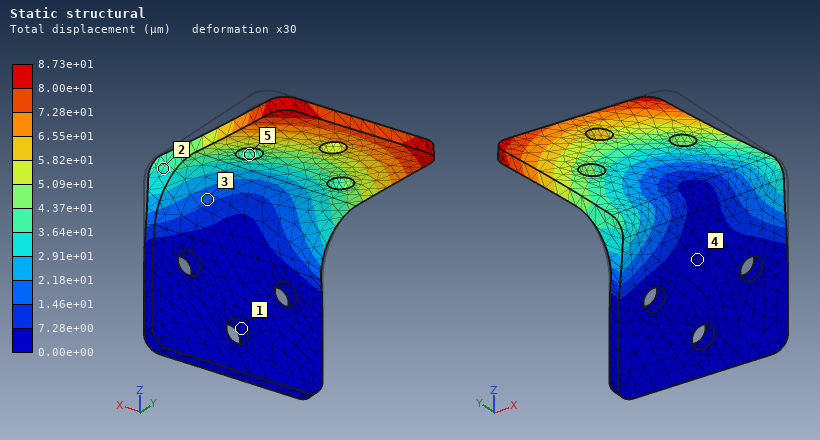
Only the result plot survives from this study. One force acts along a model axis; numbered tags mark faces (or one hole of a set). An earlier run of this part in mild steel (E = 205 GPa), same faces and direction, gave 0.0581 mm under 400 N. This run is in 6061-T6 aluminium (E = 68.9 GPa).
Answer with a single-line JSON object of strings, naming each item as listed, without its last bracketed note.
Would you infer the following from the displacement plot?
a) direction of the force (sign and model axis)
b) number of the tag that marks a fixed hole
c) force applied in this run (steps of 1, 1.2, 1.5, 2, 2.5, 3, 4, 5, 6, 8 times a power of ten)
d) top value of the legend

{"direction of the force": "-X", "number of the tag that marks a fixed hole": "1", "force applied in this run": "200 N", "top value of the legend": "8.73e+01 µm"}
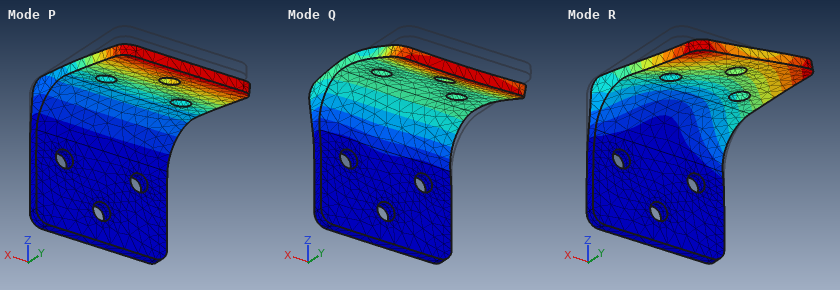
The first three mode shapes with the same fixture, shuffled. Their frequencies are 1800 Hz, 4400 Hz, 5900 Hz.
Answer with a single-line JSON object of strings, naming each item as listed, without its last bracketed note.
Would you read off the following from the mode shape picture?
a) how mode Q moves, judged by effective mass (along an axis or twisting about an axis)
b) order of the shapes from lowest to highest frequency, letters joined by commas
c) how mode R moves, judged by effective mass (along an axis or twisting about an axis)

{"how mode Q moves, judged by effective mass": "along Y", "order of the shapes from lowest to highest frequency, letters joined by commas": "P, R, Q", "how mode R moves, judged by effective mass": "along X"}
